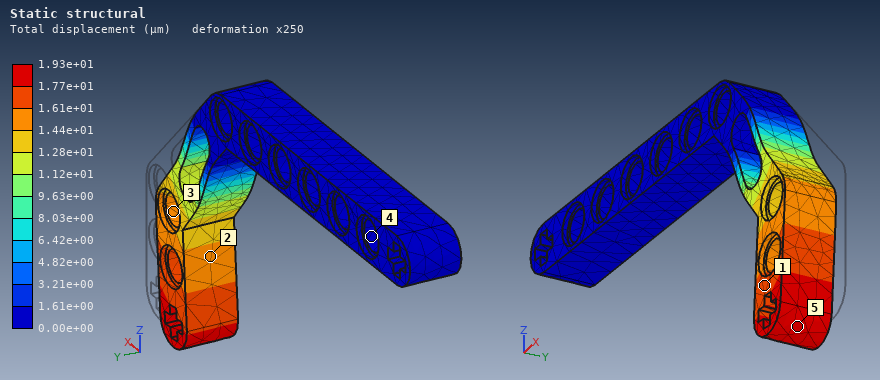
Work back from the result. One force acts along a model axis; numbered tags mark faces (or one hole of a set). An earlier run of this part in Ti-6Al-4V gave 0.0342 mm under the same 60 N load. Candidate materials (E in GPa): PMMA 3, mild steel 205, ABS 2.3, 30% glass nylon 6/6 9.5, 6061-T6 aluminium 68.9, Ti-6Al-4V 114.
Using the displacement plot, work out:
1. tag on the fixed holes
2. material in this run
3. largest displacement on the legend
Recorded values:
4
mild steel
1.93e+01 µm
